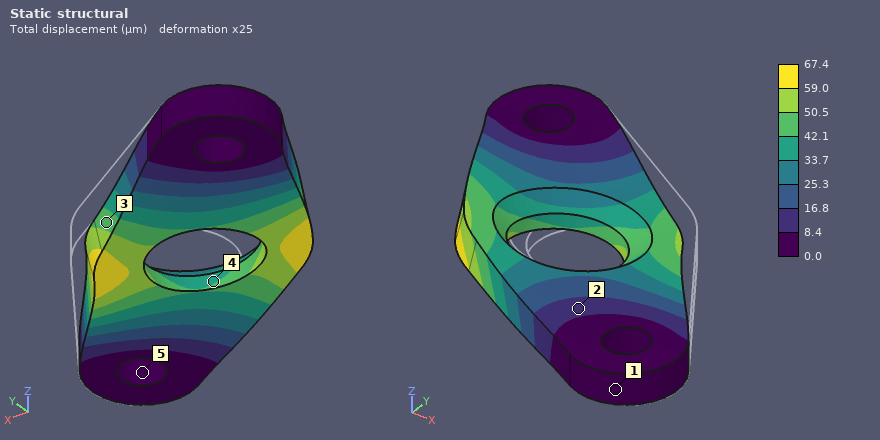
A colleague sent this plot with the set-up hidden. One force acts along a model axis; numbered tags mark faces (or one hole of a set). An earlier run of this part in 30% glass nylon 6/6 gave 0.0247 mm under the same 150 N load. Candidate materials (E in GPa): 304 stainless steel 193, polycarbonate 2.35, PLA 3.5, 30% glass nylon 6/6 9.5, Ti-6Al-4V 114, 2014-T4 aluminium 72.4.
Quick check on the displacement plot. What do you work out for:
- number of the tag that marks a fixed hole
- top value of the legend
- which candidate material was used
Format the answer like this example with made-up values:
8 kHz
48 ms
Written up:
5
67.4 µm
PLA
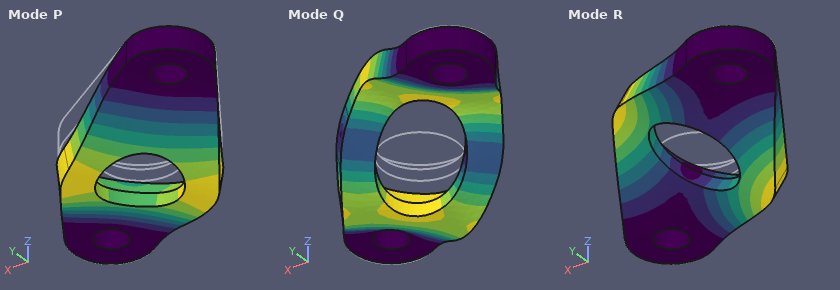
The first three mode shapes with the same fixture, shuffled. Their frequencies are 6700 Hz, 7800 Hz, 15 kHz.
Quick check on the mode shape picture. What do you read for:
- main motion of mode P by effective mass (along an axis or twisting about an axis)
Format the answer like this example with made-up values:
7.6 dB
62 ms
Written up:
along Z
